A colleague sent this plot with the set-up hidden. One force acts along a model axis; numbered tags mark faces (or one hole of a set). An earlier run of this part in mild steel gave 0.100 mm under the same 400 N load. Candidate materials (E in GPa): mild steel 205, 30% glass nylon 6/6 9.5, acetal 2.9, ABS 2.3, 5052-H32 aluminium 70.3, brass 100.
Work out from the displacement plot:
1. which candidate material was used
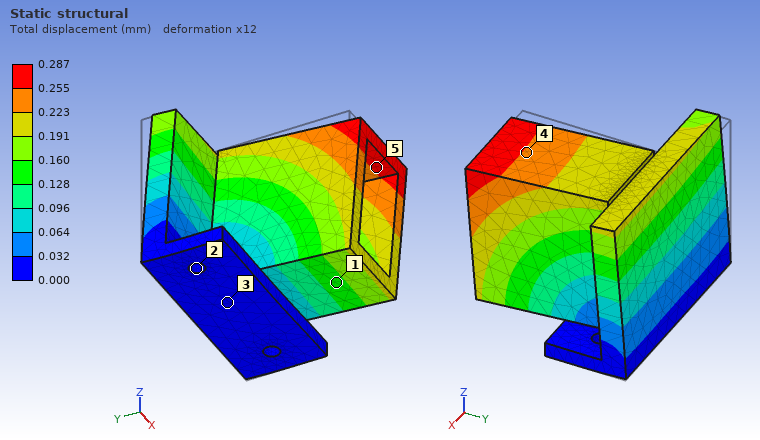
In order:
5052-H32 aluminium
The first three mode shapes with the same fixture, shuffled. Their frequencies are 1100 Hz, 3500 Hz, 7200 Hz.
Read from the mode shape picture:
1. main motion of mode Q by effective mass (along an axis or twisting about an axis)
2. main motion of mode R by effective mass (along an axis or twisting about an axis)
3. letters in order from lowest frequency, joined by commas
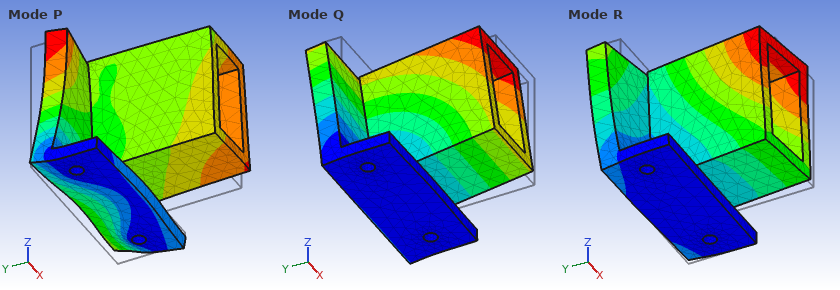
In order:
along Y
along X
Q, R, P
